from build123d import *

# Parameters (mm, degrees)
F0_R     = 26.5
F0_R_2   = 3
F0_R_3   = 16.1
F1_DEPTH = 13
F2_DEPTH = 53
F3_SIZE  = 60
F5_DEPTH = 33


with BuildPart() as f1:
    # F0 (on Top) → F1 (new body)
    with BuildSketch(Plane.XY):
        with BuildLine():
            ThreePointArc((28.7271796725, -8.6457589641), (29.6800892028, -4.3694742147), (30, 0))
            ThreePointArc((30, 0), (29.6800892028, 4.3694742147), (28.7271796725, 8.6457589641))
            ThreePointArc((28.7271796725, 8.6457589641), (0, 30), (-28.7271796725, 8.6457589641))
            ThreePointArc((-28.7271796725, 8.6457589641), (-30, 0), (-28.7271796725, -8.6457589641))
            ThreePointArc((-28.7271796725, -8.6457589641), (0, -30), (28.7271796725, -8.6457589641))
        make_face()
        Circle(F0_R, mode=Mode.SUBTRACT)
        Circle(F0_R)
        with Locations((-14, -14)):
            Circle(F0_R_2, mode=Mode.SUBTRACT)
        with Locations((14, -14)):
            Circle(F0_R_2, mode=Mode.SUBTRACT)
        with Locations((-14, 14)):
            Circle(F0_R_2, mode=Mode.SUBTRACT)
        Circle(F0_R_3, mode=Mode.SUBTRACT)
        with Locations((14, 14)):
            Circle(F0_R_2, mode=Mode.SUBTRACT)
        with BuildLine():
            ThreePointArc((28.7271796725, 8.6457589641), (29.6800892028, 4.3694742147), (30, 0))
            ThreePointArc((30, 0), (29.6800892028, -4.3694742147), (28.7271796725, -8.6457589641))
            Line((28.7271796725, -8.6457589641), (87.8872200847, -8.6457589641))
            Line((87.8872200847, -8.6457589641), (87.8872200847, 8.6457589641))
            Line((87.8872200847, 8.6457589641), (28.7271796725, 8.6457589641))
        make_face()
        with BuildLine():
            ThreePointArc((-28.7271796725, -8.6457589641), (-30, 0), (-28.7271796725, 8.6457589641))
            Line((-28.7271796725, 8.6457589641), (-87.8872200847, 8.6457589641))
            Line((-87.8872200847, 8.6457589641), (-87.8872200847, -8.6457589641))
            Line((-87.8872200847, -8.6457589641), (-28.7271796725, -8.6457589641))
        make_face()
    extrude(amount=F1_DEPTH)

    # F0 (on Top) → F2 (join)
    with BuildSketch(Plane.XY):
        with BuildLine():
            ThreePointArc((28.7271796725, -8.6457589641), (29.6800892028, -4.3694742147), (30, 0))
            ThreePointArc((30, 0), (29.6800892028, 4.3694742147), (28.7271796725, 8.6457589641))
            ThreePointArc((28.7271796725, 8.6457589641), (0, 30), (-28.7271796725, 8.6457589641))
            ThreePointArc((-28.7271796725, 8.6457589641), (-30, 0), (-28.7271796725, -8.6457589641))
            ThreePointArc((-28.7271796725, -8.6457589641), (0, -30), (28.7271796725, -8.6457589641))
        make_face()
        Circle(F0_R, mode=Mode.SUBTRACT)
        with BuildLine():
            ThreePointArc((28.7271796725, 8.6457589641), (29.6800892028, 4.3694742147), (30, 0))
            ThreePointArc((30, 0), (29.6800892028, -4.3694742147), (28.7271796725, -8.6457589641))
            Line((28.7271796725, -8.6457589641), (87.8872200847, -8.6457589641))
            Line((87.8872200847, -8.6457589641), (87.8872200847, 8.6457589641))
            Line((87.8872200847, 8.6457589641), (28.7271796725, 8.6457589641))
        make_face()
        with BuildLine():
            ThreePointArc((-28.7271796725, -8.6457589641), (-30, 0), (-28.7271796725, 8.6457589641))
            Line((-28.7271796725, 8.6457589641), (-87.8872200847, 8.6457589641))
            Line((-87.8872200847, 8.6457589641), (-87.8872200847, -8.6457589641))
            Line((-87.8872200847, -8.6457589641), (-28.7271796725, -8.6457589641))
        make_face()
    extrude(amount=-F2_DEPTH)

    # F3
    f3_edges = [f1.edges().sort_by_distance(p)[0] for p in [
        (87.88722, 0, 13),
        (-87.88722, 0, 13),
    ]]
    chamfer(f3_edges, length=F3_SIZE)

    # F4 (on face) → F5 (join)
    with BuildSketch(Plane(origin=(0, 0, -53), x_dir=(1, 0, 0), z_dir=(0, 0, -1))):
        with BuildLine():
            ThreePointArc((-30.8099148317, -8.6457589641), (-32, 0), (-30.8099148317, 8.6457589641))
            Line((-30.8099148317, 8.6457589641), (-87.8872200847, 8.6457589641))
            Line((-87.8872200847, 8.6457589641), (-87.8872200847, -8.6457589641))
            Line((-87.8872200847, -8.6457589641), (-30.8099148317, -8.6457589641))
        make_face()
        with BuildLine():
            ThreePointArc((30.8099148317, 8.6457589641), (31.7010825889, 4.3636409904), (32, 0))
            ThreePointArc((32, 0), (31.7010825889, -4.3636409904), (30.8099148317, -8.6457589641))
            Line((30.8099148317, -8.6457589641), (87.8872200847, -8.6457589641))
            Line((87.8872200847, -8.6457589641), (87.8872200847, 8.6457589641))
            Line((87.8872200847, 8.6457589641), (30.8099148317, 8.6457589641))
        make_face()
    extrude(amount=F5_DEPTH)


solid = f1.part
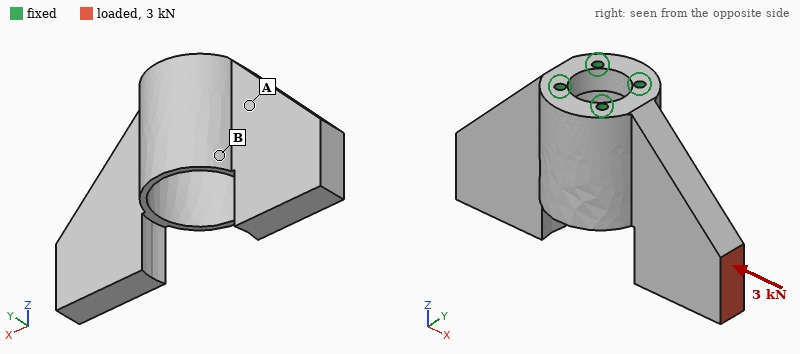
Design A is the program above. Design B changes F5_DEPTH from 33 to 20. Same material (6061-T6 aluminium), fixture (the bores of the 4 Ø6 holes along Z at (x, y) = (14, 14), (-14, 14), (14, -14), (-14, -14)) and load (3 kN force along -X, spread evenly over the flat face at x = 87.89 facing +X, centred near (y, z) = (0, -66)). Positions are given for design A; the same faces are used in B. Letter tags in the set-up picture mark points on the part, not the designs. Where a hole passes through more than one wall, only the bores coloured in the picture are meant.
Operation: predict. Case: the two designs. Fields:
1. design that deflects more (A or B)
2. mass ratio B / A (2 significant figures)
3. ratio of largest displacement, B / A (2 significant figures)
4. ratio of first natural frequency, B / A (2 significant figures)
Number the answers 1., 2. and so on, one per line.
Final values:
1. A
2. 0.87
3. 0.83
4. 1.2
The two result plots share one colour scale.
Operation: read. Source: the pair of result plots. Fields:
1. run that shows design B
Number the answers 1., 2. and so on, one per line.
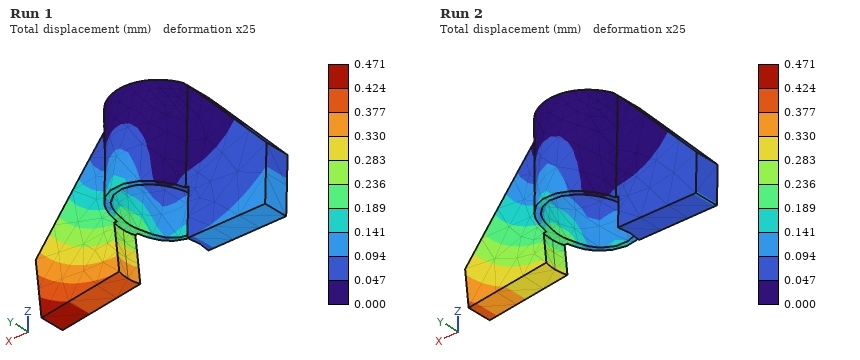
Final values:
1. Run 2
